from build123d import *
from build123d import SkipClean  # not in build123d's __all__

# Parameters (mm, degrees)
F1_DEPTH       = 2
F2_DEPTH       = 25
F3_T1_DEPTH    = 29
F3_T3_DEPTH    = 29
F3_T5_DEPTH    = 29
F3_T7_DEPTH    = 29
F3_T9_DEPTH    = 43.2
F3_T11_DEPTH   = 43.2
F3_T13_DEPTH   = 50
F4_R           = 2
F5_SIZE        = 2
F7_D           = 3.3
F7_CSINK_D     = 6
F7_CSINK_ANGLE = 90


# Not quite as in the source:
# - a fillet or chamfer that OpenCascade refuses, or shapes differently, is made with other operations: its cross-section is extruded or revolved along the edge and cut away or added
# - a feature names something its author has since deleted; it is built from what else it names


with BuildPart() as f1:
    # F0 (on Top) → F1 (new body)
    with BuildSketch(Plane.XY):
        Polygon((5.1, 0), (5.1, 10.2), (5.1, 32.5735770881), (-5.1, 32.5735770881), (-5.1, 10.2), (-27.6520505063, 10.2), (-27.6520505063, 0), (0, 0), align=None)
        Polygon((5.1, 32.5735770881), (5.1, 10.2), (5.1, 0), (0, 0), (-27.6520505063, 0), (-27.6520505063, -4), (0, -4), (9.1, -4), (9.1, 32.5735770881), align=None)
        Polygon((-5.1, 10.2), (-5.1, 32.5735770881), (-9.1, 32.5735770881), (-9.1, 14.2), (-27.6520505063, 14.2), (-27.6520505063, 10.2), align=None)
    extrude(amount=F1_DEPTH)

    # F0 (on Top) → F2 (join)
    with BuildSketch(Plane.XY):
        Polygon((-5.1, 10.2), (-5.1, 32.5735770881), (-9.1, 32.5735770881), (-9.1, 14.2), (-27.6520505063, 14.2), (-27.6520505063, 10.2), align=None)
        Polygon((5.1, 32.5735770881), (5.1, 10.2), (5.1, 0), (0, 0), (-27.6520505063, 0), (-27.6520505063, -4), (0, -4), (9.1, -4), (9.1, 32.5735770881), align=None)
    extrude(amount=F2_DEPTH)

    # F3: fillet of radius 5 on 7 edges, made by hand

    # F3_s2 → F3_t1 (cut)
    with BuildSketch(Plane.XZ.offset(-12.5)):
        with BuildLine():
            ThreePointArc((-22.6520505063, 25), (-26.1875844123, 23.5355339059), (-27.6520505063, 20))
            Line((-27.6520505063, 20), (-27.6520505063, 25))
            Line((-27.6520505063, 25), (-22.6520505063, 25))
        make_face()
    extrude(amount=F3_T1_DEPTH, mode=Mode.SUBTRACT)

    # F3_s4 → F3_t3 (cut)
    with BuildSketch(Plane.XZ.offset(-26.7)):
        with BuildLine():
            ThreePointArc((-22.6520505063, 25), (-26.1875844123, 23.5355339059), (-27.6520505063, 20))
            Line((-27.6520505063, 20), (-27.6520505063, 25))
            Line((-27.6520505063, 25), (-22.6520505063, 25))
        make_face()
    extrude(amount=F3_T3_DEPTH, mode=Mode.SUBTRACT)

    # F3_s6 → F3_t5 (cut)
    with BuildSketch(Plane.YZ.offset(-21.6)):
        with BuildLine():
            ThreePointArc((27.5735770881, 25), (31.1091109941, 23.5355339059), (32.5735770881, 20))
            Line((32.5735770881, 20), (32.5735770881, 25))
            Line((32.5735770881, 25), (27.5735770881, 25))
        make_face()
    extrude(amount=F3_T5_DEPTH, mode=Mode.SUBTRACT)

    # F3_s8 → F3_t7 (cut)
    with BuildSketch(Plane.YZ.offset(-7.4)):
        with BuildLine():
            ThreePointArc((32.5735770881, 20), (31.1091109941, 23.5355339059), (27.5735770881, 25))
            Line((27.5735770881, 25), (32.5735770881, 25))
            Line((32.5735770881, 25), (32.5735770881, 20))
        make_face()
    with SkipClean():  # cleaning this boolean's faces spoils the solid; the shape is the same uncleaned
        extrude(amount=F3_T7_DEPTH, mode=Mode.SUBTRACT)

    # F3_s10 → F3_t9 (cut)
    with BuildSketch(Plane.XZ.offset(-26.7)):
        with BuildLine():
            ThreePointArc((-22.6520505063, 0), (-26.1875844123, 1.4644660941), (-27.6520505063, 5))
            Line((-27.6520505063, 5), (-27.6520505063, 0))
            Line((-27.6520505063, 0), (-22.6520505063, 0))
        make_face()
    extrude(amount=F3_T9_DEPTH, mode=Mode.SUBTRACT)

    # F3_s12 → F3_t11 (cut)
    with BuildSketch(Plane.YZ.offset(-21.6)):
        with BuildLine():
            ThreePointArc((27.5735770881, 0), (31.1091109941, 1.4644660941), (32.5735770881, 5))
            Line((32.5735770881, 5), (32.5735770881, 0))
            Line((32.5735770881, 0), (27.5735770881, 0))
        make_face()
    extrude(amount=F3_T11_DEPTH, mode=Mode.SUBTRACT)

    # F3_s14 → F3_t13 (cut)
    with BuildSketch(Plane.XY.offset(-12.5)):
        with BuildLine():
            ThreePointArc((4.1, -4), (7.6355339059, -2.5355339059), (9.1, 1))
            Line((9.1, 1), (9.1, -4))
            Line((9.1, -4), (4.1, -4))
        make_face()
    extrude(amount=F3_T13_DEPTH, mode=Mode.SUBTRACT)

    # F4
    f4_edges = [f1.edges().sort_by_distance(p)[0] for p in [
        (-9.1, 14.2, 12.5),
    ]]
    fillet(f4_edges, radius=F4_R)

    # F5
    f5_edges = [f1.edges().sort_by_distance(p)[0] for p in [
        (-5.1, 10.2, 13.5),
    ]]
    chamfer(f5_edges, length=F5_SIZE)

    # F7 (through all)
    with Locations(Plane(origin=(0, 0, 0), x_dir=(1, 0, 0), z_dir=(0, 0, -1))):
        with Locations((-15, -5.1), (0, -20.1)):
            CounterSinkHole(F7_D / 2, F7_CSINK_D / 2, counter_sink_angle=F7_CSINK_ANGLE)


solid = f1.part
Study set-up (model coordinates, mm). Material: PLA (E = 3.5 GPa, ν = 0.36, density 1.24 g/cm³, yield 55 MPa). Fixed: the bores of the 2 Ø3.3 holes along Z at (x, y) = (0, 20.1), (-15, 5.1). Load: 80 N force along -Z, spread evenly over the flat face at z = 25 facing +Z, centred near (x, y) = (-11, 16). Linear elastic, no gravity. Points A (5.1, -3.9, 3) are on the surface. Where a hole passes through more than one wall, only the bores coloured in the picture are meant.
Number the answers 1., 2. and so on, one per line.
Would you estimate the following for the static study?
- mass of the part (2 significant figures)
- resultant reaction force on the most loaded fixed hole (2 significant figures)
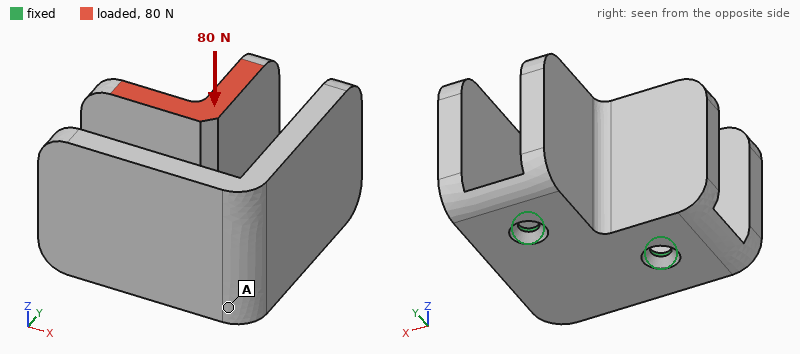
1. 14 g
2. 41 N
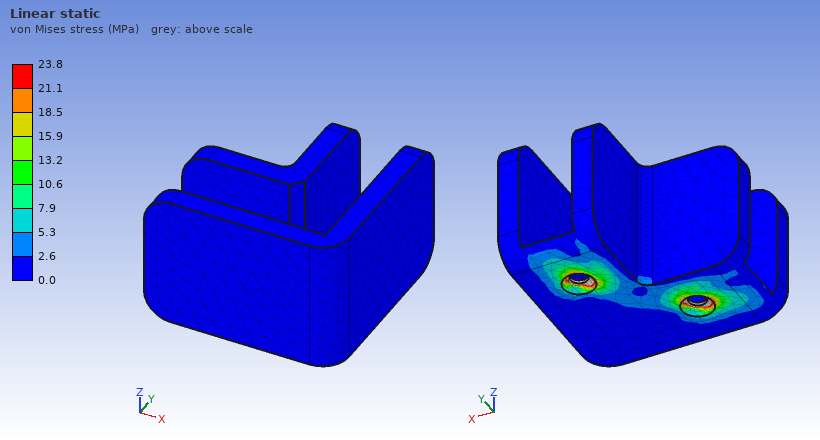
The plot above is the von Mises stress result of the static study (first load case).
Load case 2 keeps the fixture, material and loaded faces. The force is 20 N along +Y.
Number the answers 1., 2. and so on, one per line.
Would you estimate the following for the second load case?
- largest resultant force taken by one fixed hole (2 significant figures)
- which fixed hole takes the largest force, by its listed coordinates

1. 25 N
2. (0, 20.1)
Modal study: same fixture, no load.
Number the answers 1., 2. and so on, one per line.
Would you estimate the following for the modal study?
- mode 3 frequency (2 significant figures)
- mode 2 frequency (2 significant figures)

1. 920 Hz
2. 840 Hz
